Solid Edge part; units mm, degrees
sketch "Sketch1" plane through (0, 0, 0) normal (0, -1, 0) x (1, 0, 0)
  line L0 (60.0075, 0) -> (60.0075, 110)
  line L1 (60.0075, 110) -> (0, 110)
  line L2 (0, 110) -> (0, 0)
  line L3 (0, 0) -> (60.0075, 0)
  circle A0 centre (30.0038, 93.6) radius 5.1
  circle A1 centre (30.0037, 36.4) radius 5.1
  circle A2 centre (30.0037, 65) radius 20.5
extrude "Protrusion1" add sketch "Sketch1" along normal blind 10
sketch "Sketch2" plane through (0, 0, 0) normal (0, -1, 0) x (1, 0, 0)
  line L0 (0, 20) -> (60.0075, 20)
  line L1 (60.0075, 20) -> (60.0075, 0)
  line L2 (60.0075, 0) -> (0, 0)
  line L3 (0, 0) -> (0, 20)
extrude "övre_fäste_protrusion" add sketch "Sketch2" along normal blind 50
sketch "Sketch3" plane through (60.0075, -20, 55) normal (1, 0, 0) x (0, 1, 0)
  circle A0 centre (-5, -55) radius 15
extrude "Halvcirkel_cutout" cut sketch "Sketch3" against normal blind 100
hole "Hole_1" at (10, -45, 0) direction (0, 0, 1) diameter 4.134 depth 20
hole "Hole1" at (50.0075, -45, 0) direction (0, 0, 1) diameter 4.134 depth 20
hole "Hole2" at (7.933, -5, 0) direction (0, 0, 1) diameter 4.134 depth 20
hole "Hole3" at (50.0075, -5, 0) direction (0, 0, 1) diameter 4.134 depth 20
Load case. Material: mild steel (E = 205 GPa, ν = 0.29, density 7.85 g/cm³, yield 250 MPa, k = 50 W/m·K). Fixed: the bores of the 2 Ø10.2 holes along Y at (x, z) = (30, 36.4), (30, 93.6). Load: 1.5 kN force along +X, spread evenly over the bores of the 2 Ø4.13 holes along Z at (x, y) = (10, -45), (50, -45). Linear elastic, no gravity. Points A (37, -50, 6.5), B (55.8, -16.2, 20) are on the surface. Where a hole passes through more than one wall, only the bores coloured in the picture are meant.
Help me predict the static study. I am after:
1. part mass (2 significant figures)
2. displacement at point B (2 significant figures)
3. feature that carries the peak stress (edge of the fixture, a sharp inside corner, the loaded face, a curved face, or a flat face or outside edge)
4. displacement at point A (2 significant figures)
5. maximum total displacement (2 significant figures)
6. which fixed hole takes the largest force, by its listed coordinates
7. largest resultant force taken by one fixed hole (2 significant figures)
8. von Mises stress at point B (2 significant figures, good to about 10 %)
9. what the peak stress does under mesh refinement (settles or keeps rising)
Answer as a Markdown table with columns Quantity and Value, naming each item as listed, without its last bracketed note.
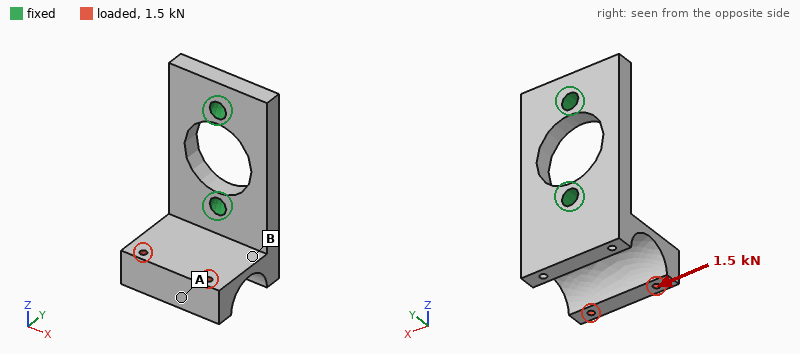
| Quantity | Value |
|---|---|
| part mass | 600 g |
| displacement at point B | 21 µm |
| feature that carries the peak stress | edge of the fixture |
| displacement at point A | 38 µm |
| maximum total displacement | 44 µm |
| which fixed hole takes the largest force, by its listed coordinates | (30, 36.4) |
| largest resultant force taken by one fixed hole | 1.7 kN |
| von Mises stress at point B | 26 MPa |
| what the peak stress does under mesh refinement | keeps rising |
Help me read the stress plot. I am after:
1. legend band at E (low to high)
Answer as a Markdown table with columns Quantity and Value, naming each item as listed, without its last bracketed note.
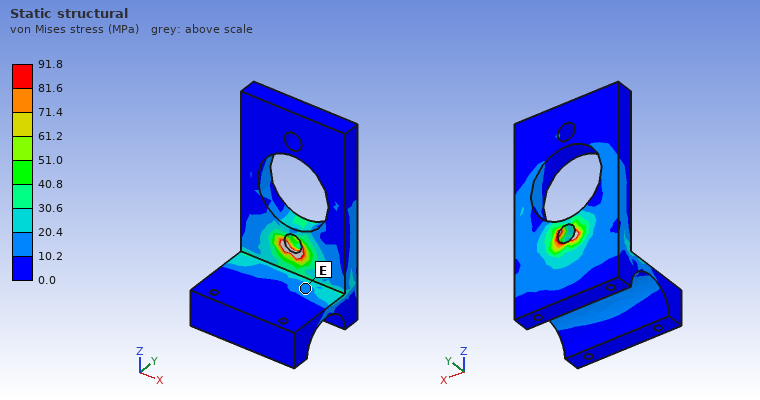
| Quantity | Value |
|---|---|
| legend band at E | 10.2 to 20.4 MPa |
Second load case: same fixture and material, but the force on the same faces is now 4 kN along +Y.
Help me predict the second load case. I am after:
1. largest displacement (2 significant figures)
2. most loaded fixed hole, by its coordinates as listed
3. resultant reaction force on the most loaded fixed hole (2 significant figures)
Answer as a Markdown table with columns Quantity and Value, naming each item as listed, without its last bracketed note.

| Quantity | Value |
|---|---|
| largest displacement | 0.17 mm |
| most loaded fixed hole, by its coordinates as listed | (30, 36.4) |
| resultant reaction force on the most loaded fixed hole | 4.3 kN |
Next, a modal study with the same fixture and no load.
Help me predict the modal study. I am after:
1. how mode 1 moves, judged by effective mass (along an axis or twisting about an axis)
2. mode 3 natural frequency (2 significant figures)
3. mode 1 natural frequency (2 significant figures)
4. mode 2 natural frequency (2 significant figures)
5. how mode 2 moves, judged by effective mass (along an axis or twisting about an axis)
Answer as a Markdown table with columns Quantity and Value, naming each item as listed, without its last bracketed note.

| Quantity | Value |
|---|---|
| how mode 1 moves, judged by effective mass | along Z |
| mode 3 natural frequency | 4300 Hz |
| mode 1 natural frequency | 1500 Hz |
| mode 2 natural frequency | 2500 Hz |
| how mode 2 moves, judged by effective mass | along X |
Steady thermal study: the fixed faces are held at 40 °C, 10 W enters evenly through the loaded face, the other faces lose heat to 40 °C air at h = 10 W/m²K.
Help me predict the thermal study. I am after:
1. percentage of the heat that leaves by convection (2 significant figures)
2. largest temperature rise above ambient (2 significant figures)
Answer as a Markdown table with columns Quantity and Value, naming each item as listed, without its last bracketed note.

| Quantity | Value |
|---|---|
| percentage of the heat that leaves by convection | 17 % |
| largest temperature rise above ambient | 24 K |
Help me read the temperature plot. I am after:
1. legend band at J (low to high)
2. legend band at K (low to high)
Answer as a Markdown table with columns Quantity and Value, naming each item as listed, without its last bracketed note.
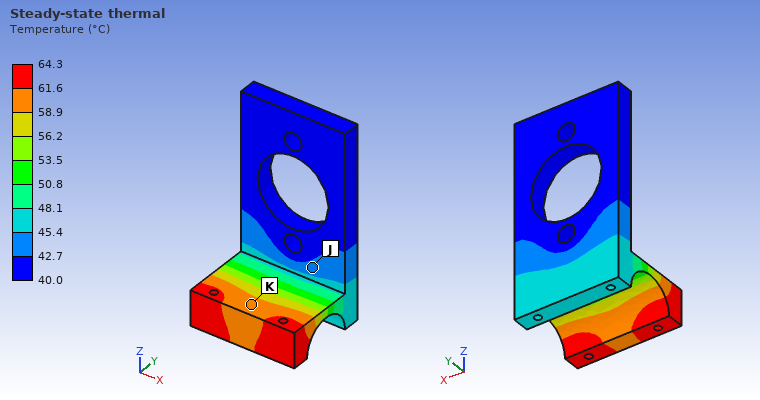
| Quantity | Value |
|---|---|
| legend band at J | 42.7 to 45.4 °C |
| legend band at K | 58.9 to 61.6 °C |
